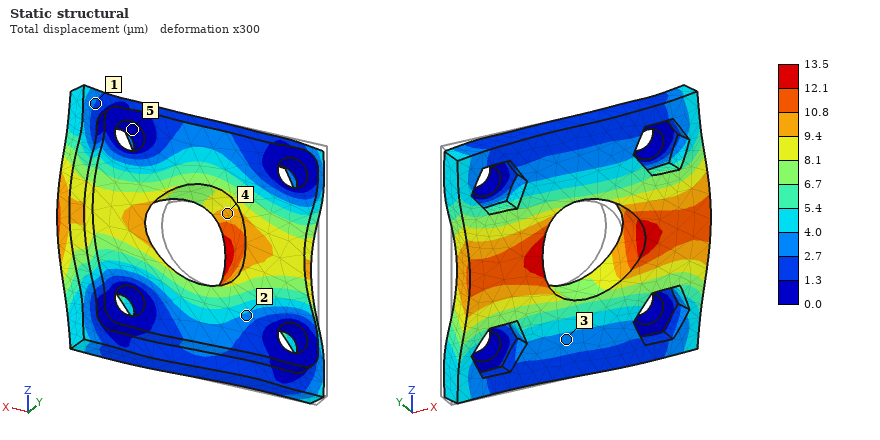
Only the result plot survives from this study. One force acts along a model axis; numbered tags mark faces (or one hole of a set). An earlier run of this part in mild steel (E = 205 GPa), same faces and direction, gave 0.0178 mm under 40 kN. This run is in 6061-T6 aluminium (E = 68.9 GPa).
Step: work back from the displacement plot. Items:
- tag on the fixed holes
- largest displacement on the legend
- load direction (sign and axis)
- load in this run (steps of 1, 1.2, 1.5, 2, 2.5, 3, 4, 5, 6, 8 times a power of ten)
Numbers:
5
13.5 µm
+X
10 kN
